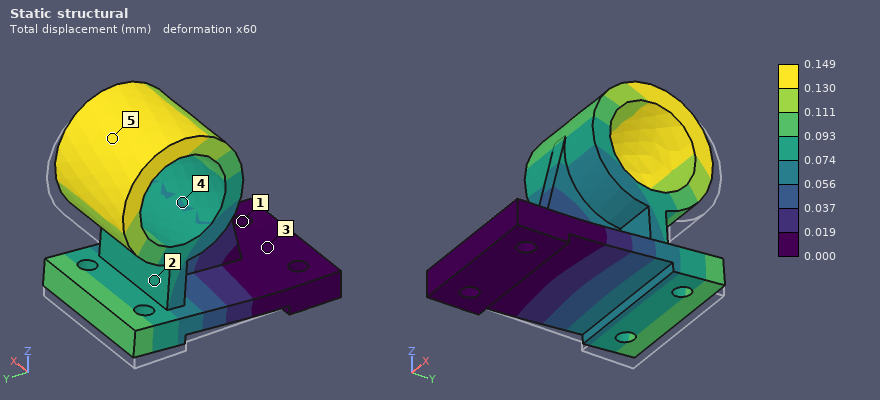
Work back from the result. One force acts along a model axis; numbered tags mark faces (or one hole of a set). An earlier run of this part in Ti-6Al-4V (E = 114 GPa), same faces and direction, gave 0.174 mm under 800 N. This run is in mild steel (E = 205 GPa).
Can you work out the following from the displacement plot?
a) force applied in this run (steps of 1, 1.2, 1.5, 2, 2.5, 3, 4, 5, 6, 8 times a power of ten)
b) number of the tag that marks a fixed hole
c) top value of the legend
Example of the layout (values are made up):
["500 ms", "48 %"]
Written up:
["1.2 kN", "1", "0.149 mm"]
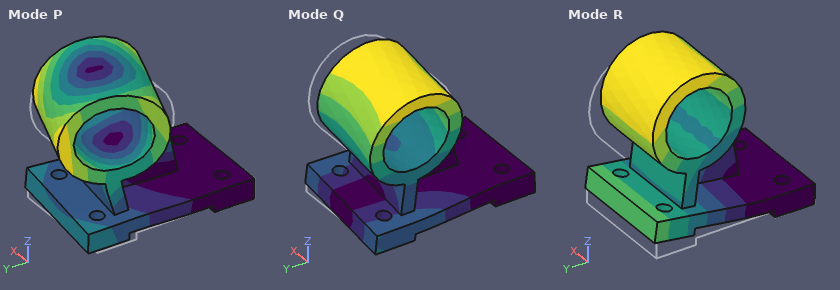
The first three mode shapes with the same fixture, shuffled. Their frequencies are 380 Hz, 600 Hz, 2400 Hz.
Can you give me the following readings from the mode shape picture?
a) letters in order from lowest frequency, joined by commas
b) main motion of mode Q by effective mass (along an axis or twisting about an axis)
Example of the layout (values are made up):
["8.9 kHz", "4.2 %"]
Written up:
["R, Q, P", "along X"]
